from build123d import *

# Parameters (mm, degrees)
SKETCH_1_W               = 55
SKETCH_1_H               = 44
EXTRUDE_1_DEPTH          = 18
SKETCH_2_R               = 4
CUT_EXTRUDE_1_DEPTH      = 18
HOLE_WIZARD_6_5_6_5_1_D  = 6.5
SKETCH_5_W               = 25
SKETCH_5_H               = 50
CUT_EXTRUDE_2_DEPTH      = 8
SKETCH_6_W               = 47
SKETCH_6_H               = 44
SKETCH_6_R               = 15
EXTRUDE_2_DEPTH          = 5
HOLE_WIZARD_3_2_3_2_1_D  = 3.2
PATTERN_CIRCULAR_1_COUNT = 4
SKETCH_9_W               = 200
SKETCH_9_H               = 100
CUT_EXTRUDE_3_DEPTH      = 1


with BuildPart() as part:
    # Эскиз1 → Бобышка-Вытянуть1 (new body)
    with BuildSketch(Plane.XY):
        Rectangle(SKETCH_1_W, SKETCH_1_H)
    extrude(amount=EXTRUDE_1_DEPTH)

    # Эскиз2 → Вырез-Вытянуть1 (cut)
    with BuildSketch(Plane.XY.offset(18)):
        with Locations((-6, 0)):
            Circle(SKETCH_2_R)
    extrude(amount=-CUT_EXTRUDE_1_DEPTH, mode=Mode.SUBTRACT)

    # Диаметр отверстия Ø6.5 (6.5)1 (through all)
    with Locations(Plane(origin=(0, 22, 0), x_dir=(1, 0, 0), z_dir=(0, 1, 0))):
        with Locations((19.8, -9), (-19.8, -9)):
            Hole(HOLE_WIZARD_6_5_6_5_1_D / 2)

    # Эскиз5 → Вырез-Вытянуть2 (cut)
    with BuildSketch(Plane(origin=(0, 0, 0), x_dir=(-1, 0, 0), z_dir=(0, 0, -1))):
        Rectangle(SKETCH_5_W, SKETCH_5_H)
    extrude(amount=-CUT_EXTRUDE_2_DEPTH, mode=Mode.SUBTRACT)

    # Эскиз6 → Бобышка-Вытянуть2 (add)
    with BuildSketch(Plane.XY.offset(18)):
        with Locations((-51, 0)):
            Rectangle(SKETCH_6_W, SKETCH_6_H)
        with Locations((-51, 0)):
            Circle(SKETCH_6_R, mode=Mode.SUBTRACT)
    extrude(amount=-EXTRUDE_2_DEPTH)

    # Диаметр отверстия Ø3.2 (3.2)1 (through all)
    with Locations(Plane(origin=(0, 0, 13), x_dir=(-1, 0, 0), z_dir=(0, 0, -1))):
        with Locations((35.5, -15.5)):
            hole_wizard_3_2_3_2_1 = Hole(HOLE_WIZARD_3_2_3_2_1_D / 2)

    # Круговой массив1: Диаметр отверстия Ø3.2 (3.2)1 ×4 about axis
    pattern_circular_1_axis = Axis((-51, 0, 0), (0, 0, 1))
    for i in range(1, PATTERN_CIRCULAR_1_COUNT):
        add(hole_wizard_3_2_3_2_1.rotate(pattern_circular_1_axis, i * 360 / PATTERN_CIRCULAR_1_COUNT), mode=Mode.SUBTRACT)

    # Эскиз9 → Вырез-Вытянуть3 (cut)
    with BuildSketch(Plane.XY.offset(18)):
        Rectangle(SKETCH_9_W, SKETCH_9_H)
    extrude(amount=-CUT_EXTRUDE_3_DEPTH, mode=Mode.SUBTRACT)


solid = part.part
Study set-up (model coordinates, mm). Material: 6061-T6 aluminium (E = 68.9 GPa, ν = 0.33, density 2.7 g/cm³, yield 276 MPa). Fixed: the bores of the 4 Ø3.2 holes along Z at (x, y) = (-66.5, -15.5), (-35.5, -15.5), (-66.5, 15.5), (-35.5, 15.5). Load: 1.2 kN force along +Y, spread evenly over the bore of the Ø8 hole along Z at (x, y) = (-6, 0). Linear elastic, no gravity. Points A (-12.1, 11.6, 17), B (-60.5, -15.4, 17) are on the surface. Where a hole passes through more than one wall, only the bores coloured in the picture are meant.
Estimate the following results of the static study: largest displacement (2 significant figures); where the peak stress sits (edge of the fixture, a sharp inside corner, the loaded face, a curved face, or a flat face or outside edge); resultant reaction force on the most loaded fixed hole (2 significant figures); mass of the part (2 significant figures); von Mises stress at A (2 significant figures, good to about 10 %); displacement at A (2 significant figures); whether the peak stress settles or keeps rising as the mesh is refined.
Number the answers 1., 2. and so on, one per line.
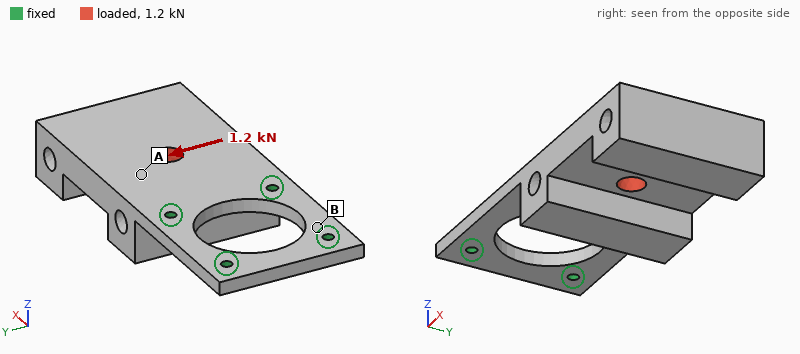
1. 24 µm
2. edge of the fixture
3. 1.2 kN
4. 93 g
5. 8.4 MPa
6. 11 µm
7. keeps rising
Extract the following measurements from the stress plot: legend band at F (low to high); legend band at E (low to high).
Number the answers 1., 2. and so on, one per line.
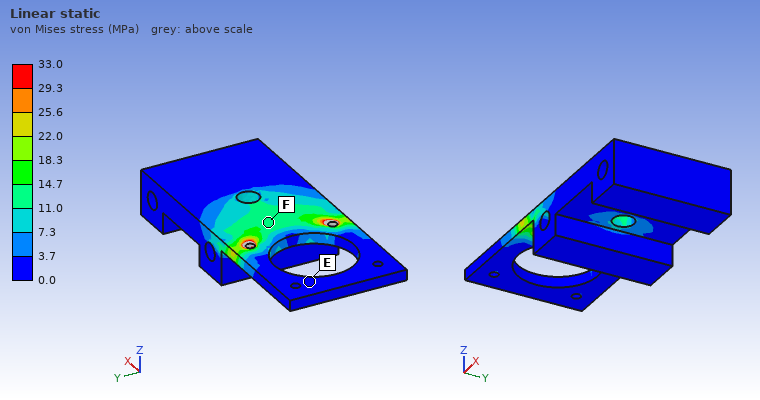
1. 11.0 to 14.7 MPa
2. 0.0 to 3.7 MPa
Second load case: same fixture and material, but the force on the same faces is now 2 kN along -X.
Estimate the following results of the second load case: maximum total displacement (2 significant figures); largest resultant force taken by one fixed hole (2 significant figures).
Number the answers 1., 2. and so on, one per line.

1. 0.22 mm
2. 1.0 kN
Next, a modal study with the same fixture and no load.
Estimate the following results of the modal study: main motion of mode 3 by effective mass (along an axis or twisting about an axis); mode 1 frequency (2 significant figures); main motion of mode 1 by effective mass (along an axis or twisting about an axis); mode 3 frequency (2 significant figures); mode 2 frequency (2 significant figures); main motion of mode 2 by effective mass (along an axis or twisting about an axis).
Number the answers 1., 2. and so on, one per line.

1. along Y
2. 550 Hz
3. along Z
4. 4300 Hz
5. 3900 Hz
6. along Y
